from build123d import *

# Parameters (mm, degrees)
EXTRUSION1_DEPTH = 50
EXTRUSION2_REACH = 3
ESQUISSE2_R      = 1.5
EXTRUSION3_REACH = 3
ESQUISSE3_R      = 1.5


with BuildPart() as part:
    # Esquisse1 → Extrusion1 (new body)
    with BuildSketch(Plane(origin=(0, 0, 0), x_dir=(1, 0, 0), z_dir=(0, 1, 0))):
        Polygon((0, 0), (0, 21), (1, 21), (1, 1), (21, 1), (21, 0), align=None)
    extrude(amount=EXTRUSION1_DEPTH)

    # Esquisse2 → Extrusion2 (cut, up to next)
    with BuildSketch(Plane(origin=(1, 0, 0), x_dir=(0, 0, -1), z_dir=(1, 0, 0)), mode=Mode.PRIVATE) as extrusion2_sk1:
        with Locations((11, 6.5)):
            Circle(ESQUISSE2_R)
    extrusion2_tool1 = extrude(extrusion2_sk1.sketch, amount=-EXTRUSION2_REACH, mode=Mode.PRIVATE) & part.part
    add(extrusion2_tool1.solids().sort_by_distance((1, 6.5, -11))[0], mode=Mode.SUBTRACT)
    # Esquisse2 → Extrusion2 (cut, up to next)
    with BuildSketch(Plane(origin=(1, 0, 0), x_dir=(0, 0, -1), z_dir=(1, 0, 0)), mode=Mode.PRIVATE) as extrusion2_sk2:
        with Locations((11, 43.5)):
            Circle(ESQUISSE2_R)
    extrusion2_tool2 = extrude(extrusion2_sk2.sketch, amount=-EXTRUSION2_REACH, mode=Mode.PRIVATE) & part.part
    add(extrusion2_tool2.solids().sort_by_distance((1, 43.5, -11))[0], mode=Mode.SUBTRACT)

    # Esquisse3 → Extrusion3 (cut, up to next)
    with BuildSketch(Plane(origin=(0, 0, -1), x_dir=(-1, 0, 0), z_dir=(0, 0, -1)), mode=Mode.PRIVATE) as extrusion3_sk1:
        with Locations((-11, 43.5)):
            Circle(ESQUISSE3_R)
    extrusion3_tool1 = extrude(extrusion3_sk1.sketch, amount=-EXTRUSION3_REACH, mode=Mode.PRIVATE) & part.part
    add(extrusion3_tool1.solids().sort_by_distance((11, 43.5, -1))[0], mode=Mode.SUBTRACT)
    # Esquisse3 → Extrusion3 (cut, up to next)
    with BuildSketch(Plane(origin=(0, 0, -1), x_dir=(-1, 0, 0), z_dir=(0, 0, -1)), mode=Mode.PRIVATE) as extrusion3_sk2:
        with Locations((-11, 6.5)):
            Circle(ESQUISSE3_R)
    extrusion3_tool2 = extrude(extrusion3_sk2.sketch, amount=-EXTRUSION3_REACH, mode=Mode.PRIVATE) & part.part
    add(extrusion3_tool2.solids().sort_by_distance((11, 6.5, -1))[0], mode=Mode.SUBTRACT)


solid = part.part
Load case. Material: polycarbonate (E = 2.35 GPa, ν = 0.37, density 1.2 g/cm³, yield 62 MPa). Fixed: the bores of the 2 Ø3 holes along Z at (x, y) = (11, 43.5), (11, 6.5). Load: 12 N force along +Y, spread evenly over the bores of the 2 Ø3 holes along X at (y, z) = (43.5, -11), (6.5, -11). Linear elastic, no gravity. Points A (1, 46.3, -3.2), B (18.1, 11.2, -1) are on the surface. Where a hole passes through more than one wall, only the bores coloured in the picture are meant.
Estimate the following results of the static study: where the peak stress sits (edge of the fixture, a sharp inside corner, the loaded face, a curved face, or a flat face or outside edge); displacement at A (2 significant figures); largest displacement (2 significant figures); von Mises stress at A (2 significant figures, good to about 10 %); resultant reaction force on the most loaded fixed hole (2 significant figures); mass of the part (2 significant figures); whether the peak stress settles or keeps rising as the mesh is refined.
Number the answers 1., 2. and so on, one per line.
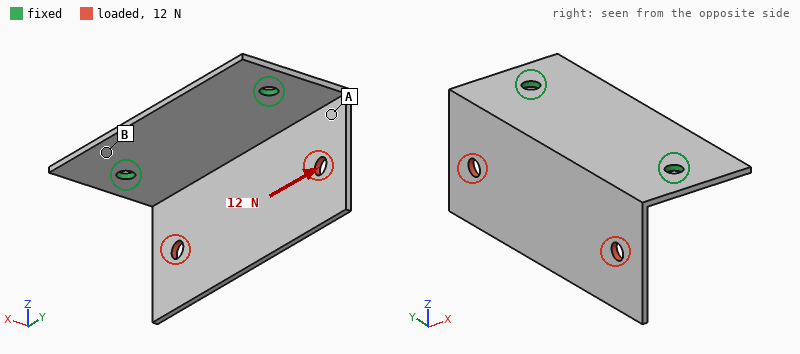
1. edge of the fixture
2. 0.25 mm
3. 0.56 mm
4. 2.9 MPa
5. 7.6 N
6. 2.4 g
7. keeps rising
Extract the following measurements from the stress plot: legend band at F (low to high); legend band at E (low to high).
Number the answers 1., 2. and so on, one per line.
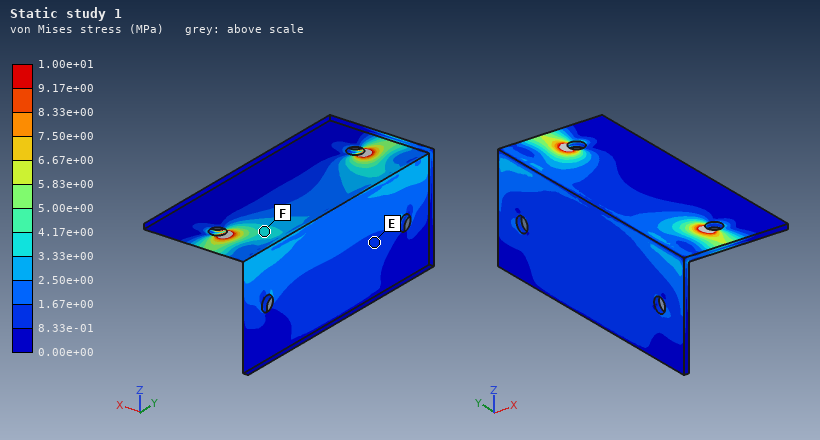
1. 3.33e+00 to 4.17e+00 MPa
2. 8.33e-01 to 1.67e+00 MPa
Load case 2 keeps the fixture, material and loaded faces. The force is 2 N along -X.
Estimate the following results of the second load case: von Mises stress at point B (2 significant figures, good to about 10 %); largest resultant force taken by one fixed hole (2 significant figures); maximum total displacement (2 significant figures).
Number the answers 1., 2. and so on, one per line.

1. 0.42 MPa
2. 1.0 N
3. 0.69 mm
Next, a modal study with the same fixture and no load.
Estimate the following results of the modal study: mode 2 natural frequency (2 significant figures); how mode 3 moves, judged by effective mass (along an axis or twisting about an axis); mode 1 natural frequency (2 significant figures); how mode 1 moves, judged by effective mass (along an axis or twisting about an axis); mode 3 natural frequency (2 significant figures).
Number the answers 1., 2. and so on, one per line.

1. 520 Hz
2. along Z
3. 290 Hz
4. along X
5. 880 Hz
